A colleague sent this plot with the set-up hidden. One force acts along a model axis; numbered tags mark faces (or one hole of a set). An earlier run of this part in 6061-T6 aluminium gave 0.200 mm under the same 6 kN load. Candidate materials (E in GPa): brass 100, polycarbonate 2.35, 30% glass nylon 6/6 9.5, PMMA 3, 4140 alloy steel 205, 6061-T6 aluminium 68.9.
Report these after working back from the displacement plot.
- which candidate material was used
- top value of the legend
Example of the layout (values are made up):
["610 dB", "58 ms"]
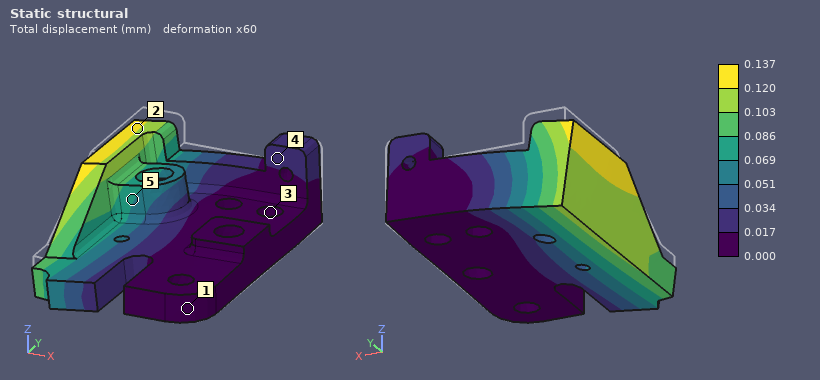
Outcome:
["brass", "0.137 mm"]
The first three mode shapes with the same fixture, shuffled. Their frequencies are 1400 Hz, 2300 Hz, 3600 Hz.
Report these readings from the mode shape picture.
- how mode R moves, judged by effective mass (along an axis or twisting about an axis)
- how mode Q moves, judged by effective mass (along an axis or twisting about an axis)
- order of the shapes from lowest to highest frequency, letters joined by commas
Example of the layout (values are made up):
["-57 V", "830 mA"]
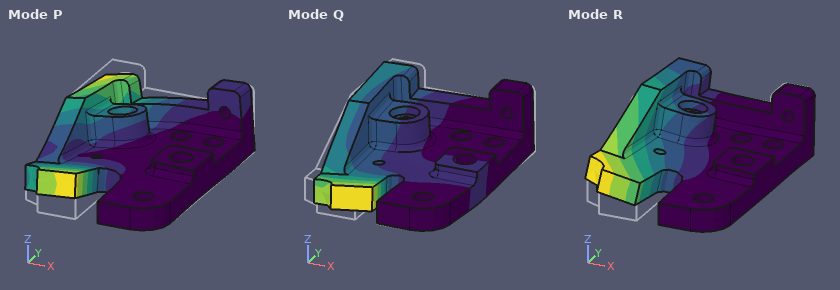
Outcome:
["along Z", "along Y", "R, P, Q"]
